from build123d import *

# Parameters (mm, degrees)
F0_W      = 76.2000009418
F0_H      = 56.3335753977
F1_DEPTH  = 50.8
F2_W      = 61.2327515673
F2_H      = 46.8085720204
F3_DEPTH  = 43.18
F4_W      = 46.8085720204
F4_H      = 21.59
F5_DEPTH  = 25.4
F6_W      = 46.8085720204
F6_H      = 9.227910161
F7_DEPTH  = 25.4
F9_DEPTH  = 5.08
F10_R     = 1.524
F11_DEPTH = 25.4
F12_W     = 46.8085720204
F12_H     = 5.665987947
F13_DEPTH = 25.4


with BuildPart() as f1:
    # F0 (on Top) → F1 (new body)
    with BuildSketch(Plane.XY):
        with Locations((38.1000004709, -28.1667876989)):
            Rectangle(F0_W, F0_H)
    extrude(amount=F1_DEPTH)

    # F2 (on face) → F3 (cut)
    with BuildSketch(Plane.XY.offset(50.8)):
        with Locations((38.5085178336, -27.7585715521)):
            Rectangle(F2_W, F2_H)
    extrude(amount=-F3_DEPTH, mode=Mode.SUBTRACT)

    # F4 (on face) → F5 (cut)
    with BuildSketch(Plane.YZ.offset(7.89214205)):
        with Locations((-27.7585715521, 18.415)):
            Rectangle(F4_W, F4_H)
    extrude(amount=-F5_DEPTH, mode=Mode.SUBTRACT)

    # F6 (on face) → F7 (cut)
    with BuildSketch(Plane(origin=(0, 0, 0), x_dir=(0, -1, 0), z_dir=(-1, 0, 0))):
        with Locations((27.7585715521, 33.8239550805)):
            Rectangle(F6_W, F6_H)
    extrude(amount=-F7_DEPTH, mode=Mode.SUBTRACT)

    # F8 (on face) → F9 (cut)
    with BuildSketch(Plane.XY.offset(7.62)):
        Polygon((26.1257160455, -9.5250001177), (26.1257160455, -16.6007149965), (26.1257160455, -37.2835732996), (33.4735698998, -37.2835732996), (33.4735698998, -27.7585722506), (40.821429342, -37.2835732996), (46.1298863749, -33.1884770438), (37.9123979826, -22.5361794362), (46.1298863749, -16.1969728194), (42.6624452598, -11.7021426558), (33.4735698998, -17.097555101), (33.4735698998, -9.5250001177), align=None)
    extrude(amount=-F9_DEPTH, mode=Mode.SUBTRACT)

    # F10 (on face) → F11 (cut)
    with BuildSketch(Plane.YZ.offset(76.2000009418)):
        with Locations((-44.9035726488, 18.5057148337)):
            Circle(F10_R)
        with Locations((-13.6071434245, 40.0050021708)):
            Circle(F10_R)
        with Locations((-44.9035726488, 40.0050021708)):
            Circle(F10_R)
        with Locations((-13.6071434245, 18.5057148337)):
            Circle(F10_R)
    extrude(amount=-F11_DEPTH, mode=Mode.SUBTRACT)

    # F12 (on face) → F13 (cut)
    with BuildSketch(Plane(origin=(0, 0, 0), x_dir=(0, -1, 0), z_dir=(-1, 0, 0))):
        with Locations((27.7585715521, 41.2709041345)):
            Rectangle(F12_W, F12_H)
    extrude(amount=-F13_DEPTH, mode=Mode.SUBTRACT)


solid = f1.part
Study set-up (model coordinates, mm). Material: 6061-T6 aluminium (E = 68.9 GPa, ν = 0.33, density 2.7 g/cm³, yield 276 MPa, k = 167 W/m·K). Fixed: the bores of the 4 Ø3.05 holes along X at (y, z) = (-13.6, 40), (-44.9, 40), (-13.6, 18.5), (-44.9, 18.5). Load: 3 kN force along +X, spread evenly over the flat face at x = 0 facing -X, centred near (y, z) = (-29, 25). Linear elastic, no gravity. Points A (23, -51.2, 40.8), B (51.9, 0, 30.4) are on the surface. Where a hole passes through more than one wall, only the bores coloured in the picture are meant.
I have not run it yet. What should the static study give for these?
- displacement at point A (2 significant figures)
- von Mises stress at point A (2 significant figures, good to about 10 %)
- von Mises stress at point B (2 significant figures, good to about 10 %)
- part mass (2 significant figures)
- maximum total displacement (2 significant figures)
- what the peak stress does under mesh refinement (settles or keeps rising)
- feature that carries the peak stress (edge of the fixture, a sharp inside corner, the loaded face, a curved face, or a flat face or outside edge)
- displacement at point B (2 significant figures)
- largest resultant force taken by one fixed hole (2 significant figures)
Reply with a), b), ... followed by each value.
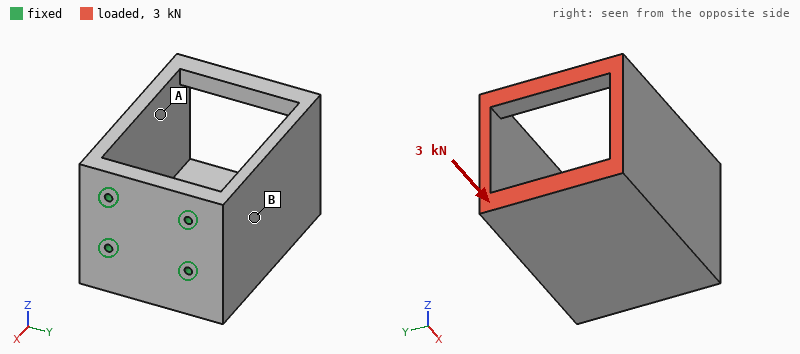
a) 18 µm
b) 16 MPa
c) 7.5 MPa
d) 210 g
e) 68 µm
f) keeps rising
g) edge of the fixture
h) 16 µm
i) 1.0 kN
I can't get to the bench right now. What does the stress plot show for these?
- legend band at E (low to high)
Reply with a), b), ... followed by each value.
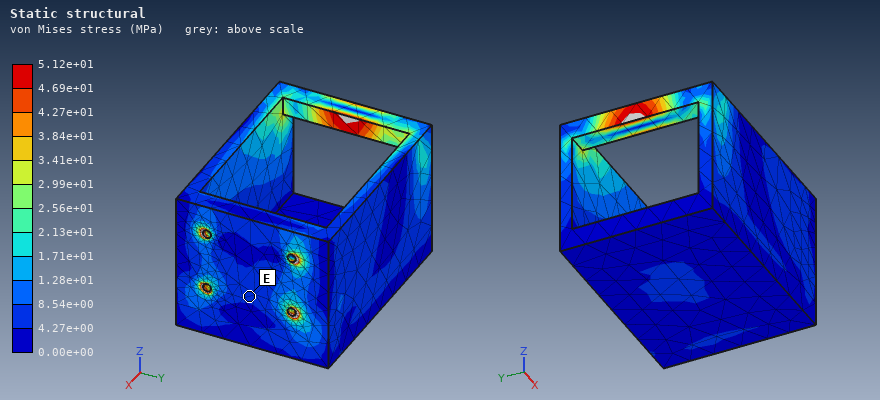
a) 4.27e+00 to 8.54e+00 MPa
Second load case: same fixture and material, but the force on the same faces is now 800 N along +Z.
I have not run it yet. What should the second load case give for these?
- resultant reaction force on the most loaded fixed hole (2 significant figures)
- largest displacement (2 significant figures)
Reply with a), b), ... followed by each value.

a) 1.2 kN
b) 85 µm
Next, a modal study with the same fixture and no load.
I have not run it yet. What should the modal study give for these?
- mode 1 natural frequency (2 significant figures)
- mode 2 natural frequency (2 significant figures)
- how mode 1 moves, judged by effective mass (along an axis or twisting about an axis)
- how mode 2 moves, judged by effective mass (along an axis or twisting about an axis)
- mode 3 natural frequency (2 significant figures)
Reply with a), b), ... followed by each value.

a) 1500 Hz
b) 2200 Hz
c) along Y
d) along Z
e) 3700 Hz
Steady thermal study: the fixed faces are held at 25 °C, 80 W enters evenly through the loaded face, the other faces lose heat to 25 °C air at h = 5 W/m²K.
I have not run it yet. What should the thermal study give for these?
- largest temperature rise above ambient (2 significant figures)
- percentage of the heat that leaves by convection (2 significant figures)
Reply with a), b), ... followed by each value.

a) 75 K
b) 4.6 %
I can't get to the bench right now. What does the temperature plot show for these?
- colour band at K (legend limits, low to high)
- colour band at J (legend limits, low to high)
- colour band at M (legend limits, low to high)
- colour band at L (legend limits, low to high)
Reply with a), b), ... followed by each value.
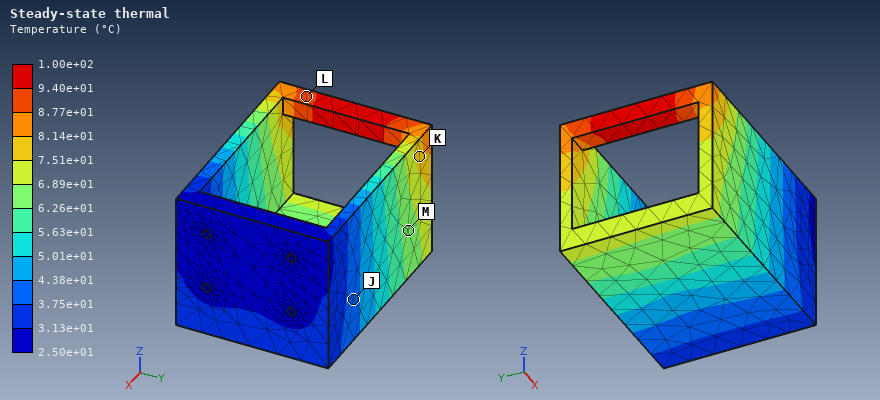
a) 7.51e+01 to 8.14e+01 °C
b) 3.75e+01 to 4.38e+01 °C
c) 6.26e+01 to 6.89e+01 °C
d) 8.77e+01 to 9.40e+01 °C
